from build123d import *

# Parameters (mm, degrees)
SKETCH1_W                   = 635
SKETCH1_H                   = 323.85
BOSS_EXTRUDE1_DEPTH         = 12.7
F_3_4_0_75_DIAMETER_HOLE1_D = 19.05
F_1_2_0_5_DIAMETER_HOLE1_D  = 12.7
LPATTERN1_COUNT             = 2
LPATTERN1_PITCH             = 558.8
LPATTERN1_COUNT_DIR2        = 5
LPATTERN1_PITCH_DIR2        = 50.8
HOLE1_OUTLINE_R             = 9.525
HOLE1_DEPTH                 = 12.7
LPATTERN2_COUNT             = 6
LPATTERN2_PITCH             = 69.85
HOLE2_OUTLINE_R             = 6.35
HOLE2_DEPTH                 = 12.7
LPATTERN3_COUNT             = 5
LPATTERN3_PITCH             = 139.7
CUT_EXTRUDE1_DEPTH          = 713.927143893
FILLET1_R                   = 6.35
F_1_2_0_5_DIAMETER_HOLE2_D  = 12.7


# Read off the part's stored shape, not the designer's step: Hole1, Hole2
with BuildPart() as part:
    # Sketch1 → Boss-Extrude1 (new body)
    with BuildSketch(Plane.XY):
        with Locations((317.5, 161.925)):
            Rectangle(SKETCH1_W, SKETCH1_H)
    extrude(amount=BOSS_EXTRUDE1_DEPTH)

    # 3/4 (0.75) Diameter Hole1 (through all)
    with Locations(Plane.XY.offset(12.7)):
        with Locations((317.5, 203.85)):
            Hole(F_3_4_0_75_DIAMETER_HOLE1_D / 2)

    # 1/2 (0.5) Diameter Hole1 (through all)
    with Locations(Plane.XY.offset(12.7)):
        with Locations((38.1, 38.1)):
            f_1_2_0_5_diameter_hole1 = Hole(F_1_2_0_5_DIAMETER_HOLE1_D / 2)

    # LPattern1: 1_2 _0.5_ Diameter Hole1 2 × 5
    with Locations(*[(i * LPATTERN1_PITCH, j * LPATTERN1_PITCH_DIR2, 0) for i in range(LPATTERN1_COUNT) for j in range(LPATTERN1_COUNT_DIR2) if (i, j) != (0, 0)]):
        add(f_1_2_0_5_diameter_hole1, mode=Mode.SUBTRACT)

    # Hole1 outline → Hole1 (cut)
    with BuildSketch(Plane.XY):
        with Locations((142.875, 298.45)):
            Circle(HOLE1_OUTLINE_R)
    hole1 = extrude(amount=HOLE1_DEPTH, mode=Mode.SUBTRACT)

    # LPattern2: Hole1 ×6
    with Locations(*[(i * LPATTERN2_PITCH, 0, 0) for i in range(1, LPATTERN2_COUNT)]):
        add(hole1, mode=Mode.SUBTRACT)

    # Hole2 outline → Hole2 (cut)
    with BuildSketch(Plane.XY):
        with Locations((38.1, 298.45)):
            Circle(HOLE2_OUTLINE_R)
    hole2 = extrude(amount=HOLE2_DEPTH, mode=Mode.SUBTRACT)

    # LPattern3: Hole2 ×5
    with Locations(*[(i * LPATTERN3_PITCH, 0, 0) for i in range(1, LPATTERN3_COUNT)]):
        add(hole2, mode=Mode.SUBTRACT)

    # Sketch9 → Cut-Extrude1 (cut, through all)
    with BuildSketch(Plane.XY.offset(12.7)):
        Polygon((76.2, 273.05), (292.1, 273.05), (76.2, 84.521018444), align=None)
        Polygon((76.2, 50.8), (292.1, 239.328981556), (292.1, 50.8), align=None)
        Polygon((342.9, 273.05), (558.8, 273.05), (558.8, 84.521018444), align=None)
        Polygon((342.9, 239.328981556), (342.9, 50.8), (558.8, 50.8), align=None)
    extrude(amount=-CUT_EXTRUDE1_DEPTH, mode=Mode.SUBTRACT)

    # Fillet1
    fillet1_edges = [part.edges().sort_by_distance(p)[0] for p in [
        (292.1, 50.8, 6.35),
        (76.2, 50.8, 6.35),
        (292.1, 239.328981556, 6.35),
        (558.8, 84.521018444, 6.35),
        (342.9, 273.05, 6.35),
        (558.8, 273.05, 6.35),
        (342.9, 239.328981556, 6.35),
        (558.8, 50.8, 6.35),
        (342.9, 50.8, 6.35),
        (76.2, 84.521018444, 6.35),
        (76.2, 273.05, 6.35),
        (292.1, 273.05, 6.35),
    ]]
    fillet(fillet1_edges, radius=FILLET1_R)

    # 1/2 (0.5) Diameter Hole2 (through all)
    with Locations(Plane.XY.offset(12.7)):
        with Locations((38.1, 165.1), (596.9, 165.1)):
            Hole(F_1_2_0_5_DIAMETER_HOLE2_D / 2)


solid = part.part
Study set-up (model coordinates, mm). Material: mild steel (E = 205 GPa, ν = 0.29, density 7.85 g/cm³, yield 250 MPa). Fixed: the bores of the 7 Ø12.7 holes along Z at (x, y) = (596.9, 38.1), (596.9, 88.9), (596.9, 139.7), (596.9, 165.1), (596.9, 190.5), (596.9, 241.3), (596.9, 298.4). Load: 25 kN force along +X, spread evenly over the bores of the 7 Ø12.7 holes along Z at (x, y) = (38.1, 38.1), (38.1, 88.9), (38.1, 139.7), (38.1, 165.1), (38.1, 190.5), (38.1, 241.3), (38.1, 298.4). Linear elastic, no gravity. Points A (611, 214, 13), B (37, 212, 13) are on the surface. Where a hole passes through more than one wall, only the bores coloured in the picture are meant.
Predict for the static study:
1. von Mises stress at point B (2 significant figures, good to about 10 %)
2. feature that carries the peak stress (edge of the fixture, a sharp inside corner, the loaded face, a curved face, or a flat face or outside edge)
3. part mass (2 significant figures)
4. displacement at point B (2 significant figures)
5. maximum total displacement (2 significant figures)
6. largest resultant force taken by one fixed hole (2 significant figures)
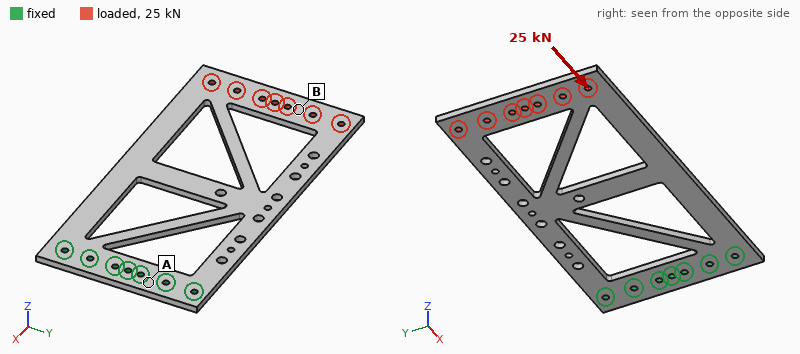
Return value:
16 MPa
a curved face
12 kg
0.10 mm
0.11 mm
12 kN
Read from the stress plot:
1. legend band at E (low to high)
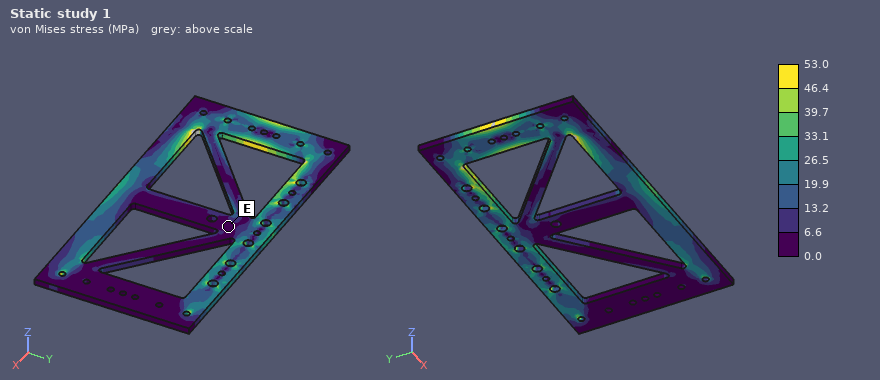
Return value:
0.0 to 6.6 MPa
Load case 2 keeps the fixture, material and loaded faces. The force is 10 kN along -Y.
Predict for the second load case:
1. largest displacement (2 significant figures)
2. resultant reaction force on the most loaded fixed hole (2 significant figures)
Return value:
0.34 mm
22 kN
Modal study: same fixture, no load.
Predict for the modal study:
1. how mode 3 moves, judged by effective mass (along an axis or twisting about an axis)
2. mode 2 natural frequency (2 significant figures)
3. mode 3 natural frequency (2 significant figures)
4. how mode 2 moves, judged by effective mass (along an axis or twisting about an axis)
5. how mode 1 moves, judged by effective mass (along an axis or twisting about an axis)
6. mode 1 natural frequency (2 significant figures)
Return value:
along Z
88 Hz
140 Hz
twisting about X
along Z
23 Hz
